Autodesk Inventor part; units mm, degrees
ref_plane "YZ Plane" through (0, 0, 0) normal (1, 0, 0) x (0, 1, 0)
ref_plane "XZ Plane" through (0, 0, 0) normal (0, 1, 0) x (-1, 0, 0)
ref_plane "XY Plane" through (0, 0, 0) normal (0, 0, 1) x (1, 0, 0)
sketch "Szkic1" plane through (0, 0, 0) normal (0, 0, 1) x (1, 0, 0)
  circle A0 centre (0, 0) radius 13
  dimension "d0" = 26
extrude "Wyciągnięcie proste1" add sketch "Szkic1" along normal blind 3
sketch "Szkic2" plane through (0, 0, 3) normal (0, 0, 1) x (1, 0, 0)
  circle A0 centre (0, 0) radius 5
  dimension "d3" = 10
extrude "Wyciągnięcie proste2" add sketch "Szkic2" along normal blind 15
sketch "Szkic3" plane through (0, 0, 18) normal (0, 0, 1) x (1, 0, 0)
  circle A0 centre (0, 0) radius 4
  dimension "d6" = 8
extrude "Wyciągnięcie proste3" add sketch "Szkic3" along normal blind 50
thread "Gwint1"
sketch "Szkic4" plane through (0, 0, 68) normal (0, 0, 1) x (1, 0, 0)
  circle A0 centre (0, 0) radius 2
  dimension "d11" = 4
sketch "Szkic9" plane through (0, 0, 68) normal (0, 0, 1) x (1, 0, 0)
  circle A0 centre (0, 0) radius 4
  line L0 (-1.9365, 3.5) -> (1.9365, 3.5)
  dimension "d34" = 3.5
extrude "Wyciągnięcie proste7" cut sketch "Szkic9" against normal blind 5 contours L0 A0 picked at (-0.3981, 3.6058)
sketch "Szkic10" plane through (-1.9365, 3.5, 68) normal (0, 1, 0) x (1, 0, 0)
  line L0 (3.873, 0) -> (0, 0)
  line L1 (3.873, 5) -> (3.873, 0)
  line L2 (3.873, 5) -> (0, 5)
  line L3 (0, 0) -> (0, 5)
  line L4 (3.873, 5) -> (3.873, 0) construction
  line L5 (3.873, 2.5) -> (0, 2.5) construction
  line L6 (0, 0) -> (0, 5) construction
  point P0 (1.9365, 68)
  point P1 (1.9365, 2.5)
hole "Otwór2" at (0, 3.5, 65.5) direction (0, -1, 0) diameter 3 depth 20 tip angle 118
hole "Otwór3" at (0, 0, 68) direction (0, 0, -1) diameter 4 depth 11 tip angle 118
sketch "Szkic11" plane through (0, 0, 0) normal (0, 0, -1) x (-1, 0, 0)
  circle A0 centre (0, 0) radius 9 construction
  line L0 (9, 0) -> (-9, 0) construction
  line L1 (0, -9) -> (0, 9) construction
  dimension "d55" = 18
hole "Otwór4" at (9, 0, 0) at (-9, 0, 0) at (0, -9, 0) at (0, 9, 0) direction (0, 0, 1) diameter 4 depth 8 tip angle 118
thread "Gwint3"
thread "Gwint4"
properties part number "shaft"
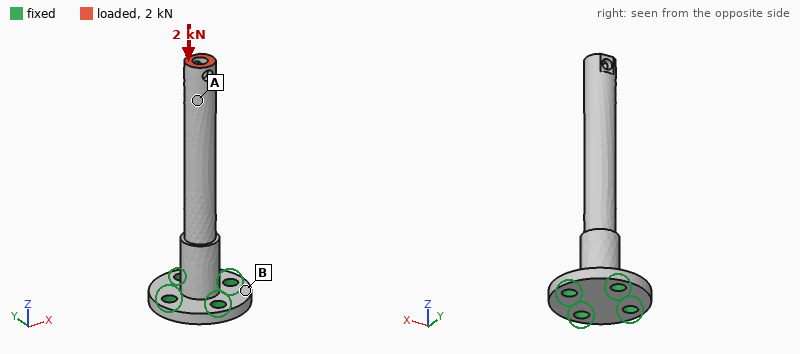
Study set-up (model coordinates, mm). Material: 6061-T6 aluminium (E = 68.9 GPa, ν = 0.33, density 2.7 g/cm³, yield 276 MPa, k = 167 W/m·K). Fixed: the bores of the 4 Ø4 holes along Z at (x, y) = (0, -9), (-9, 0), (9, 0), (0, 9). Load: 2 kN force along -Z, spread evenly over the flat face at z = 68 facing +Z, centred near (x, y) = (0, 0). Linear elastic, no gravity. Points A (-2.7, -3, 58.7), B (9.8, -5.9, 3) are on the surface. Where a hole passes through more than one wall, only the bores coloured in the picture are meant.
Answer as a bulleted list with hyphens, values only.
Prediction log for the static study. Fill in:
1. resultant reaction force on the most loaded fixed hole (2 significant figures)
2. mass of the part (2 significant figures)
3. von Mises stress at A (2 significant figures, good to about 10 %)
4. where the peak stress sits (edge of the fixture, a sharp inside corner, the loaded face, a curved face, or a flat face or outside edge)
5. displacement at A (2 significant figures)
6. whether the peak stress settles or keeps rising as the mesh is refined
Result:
- 540 N
- 13 g
- 56 MPa
- a sharp inside corner
- 46 µm
- keeps rising
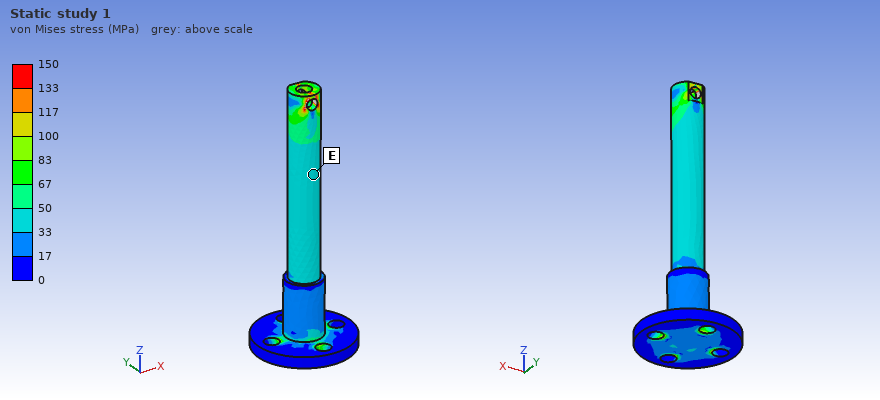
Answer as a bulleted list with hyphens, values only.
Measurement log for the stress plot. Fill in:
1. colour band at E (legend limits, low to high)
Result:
- 33 to 50 MPa
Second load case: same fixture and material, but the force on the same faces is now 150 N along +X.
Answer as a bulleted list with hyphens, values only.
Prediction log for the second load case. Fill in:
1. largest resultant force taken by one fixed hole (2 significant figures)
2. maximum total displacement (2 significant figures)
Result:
- 680 N
- 0.78 mm
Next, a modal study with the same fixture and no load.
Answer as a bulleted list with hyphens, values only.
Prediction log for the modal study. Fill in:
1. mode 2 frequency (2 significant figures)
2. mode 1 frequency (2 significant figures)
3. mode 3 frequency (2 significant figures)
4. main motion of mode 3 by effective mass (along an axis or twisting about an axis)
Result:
- 1700 Hz
- 1700 Hz
- 8500 Hz
- along X
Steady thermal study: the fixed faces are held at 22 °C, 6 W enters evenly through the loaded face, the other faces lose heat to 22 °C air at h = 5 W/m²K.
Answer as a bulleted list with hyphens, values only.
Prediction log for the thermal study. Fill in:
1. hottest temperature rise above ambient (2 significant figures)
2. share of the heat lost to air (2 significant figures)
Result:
- 49 K
- 3.6 %
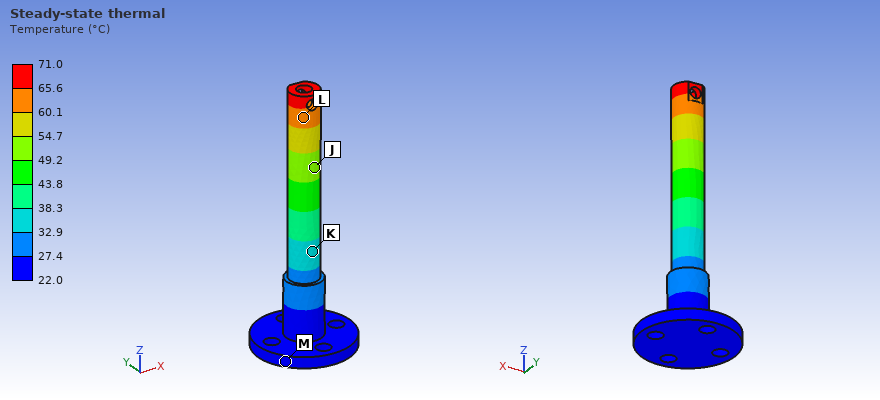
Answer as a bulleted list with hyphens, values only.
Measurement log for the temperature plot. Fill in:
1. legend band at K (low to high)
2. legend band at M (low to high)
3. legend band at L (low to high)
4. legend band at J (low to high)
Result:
- 32.9 to 38.3 °C
- 22.0 to 27.4 °C
- 60.1 to 65.6 °C
- 49.2 to 54.7 °C
